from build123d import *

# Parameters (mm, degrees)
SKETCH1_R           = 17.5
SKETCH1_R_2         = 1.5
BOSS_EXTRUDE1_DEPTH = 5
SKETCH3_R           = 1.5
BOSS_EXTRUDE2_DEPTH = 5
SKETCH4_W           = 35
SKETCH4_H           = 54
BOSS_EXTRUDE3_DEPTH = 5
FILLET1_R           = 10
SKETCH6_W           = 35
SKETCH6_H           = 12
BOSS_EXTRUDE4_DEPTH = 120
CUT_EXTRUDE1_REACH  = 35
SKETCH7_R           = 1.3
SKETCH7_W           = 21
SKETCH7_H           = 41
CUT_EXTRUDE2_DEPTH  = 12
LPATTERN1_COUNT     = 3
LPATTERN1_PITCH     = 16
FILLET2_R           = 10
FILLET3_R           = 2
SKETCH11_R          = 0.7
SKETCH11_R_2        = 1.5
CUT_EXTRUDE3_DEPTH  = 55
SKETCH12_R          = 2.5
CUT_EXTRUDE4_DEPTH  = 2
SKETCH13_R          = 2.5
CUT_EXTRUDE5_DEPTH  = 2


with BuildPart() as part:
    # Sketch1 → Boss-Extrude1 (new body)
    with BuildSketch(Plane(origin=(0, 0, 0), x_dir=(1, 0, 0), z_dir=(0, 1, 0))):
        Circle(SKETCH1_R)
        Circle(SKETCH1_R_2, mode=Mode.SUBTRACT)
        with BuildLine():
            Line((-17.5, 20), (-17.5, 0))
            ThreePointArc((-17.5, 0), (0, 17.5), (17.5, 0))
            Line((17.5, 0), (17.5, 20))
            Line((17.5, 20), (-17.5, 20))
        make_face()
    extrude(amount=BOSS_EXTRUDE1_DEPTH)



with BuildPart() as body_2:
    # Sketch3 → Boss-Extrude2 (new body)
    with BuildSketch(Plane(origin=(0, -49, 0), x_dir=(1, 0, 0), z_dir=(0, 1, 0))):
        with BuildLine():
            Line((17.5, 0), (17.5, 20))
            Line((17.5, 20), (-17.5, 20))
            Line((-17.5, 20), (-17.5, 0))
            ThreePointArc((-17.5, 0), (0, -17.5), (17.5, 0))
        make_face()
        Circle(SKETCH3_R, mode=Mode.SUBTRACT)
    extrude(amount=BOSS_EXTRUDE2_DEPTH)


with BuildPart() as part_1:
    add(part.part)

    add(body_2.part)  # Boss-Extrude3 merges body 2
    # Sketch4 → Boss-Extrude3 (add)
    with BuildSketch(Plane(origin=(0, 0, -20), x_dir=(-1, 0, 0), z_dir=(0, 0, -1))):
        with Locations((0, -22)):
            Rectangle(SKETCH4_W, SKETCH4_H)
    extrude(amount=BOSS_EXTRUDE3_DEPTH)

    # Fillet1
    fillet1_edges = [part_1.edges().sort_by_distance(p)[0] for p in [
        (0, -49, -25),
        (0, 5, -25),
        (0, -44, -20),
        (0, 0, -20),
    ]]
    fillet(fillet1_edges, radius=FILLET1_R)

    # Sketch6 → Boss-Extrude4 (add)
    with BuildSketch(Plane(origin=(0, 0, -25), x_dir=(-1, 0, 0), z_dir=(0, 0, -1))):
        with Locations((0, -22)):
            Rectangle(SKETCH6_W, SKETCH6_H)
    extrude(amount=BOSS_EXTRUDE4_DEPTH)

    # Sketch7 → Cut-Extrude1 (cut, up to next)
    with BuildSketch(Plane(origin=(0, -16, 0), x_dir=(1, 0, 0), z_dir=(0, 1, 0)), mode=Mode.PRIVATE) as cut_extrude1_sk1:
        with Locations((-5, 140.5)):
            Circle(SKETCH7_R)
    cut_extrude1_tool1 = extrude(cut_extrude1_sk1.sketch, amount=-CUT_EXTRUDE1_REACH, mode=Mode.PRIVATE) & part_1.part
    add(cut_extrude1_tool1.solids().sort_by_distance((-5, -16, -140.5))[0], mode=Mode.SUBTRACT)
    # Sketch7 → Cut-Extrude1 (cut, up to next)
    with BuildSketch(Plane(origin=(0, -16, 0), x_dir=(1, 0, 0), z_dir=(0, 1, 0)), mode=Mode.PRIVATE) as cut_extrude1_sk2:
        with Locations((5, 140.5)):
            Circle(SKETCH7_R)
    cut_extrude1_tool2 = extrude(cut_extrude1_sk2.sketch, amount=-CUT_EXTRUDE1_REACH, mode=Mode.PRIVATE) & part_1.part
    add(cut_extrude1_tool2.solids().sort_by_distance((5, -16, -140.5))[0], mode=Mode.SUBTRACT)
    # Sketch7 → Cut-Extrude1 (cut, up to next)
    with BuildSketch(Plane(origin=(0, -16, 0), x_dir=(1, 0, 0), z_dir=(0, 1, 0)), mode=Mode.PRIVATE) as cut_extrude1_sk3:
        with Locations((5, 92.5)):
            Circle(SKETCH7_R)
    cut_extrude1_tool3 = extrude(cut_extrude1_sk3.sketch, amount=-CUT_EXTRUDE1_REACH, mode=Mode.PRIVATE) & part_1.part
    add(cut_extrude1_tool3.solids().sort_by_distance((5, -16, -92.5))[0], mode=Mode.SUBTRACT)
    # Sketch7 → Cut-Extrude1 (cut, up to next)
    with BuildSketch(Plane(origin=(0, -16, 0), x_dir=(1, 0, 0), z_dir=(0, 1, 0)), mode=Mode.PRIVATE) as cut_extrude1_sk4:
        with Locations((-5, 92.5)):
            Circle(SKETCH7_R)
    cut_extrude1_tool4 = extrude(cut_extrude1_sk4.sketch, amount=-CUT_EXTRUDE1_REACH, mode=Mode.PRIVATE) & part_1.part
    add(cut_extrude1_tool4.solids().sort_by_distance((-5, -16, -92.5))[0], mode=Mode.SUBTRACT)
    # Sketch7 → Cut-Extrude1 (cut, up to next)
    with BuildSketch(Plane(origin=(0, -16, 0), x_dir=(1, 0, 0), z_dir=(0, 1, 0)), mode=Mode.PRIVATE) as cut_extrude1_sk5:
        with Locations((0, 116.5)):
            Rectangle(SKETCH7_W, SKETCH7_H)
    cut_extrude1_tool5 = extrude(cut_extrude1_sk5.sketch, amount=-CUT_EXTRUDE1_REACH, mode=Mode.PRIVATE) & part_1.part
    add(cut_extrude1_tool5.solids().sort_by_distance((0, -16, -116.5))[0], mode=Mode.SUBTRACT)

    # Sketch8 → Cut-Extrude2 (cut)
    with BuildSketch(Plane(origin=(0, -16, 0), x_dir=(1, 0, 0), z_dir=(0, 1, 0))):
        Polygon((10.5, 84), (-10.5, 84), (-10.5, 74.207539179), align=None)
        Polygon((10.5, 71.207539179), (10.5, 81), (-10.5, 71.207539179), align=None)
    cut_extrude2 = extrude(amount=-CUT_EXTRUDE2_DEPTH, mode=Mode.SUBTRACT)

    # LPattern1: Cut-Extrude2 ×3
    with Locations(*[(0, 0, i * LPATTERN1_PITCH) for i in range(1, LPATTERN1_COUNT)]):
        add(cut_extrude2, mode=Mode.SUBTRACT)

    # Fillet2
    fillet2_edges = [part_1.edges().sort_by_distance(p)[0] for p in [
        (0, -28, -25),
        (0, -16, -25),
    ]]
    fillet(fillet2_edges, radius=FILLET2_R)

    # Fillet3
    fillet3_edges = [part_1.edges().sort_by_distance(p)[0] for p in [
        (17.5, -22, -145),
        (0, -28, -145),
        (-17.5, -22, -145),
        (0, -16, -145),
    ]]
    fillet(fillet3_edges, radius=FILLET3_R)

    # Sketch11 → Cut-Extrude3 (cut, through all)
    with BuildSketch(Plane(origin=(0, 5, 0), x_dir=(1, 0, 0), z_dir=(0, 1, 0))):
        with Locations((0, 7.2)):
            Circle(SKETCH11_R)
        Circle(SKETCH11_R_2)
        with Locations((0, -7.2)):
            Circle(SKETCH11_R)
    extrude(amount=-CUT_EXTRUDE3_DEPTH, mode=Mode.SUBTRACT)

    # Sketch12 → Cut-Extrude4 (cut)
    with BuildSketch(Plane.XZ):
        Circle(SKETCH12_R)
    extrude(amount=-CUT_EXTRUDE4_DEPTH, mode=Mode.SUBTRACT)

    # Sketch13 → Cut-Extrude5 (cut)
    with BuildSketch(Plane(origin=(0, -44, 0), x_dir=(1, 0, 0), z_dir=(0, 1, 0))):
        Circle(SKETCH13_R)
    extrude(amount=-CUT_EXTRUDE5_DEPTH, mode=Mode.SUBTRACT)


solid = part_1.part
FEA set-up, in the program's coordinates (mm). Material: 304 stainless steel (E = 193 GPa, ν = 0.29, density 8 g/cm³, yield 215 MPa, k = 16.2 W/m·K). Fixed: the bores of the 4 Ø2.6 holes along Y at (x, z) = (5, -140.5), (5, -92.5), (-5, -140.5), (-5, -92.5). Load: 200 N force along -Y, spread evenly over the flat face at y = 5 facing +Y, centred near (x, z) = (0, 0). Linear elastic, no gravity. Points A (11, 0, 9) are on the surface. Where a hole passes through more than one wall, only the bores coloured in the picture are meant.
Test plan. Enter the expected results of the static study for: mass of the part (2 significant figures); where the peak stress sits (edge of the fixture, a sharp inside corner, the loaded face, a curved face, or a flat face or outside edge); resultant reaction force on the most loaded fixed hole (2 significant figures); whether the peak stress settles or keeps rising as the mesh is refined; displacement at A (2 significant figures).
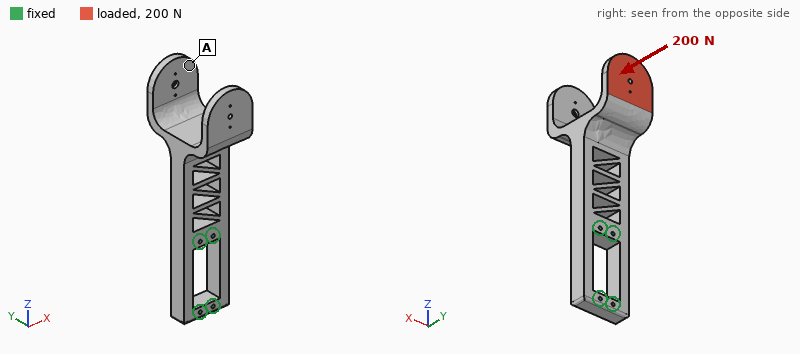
440 g
edge of the fixture
170 N
keeps rising
0.18 mm
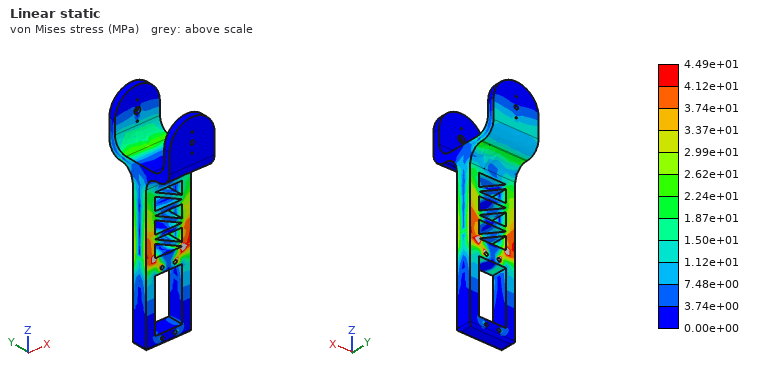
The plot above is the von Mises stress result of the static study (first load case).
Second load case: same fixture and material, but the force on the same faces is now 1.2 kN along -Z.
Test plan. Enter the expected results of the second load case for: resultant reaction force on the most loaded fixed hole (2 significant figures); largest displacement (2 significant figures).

570 N
0.52 mm
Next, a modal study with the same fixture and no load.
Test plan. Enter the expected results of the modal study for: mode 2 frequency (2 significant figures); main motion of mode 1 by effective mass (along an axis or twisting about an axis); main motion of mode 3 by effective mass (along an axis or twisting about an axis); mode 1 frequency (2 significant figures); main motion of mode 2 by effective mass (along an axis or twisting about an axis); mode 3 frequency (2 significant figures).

1200 Hz
along Y
twisting about Z
480 Hz
along X
1400 Hz
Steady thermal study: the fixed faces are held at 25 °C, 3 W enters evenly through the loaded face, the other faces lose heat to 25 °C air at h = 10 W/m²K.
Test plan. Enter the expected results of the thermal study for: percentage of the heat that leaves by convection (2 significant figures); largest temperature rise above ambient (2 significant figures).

80 %
44 K
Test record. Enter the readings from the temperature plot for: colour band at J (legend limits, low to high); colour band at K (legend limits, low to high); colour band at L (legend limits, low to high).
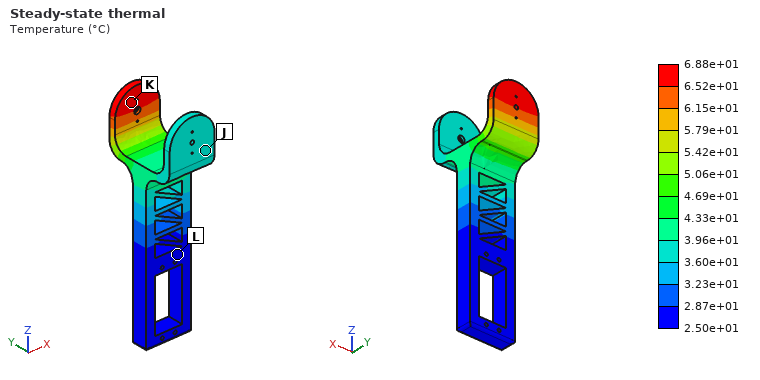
3.60e+01 to 3.96e+01 °C
6.52e+01 to 6.88e+01 °C
2.50e+01 to 2.87e+01 °C
